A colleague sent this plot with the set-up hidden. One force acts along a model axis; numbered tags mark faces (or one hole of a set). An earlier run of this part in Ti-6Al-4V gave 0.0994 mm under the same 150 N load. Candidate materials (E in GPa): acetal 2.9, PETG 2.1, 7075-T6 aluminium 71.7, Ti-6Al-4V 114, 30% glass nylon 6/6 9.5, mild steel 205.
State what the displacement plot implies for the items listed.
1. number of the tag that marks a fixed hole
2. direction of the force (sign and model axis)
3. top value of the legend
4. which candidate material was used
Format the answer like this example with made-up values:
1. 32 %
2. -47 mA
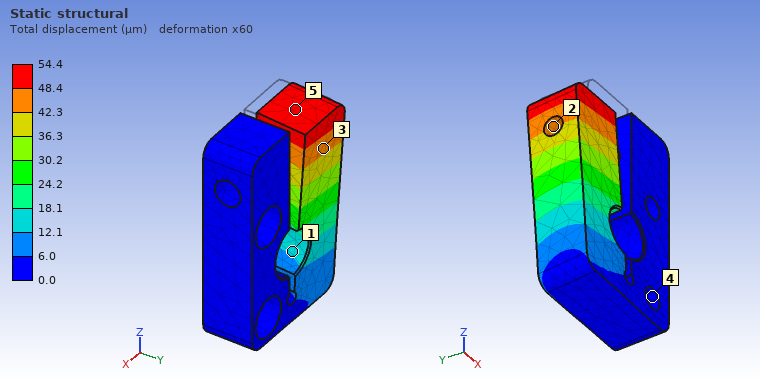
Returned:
1. 4
2. +Y
3. 54.4 µm
4. mild steel
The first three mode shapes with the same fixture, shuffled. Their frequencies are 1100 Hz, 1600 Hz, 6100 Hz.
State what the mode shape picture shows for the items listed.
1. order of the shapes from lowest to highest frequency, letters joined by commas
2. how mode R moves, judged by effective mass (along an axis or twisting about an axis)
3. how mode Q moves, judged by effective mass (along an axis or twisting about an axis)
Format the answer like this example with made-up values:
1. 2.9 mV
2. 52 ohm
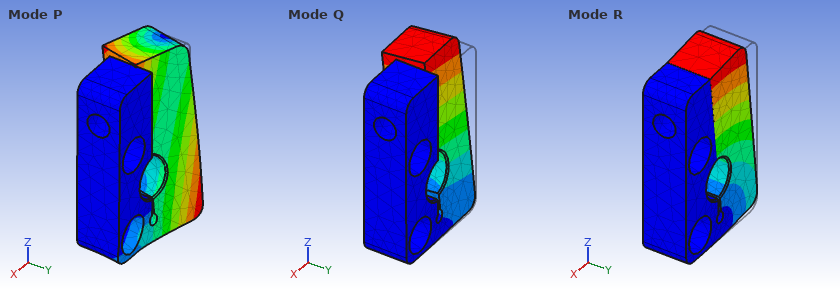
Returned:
1. R, Q, P
2. along X
3. along Y
